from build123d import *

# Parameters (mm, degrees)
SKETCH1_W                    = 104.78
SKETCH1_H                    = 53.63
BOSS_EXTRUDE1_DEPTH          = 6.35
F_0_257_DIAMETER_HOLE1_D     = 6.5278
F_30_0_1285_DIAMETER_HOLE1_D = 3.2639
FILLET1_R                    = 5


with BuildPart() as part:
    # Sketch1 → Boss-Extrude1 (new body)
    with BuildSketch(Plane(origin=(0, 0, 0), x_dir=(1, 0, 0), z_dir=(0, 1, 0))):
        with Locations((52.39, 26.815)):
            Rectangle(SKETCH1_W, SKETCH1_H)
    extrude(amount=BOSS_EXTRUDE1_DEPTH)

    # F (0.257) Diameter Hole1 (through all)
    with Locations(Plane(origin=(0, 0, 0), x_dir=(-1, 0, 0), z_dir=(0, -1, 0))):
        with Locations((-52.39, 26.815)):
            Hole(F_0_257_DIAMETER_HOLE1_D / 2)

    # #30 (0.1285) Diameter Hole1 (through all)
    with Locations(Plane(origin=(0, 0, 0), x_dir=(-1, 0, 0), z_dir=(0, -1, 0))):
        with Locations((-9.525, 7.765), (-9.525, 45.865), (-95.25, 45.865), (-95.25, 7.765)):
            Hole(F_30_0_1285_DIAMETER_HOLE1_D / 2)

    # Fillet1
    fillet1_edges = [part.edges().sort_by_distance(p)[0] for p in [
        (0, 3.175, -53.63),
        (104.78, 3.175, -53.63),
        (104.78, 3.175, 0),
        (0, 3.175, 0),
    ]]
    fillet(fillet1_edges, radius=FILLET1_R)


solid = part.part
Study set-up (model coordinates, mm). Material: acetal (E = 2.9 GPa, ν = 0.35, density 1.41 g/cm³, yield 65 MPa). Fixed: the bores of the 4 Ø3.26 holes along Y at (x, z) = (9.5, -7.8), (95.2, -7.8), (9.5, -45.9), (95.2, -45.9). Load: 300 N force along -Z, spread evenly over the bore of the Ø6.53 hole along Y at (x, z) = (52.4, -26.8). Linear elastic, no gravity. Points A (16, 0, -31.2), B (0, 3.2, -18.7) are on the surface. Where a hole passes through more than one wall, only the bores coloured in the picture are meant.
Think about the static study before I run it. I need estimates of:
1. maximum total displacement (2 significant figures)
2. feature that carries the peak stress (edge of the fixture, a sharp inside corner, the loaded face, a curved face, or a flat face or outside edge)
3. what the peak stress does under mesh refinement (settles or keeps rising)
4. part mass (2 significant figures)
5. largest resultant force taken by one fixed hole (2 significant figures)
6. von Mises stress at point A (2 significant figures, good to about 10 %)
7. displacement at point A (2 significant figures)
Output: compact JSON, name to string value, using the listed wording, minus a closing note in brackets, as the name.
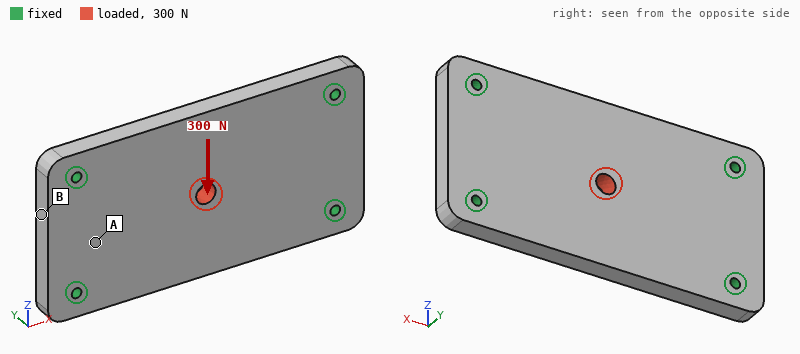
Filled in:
{"maximum total displacement": "30 µm", "feature that carries the peak stress": "edge of the fixture", "what the peak stress does under mesh refinement": "keeps rising", "part mass": "50 g", "largest resultant force taken by one fixed hole": "110 N", "von Mises stress at point A": "0.85 MPa", "displacement at point A": "5.2 µm"}
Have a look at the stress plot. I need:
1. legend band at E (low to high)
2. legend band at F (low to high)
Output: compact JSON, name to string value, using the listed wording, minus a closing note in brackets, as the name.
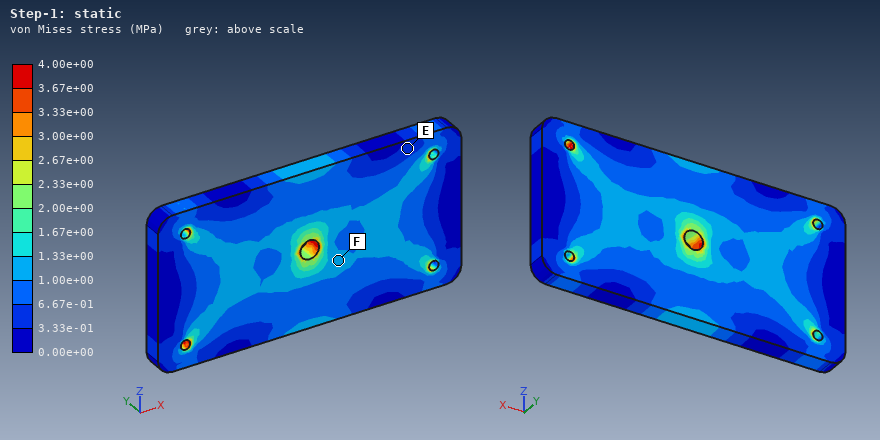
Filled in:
{"legend band at E": "3.33e-01 to 6.67e-01 MPa", "legend band at F": "1.00e+00 to 1.33e+00 MPa"}
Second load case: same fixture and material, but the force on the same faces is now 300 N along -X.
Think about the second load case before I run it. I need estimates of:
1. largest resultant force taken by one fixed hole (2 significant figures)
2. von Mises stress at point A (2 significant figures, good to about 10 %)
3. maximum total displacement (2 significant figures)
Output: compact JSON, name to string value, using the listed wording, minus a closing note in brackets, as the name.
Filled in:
{"largest resultant force taken by one fixed hole": "77 N", "von Mises stress at point A": "0.27 MPa", "maximum total displacement": "15 µm"}
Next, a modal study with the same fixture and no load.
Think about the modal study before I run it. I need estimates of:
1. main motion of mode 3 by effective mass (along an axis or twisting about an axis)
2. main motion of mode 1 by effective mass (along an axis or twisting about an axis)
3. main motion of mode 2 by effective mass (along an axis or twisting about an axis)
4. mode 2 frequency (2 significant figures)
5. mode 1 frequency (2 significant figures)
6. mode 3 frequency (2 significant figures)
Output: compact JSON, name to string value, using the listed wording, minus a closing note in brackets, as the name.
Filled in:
{"main motion of mode 3 by effective mass": "twisting about Z", "main motion of mode 1 by effective mass": "along Y", "main motion of mode 2 by effective mass": "twisting about X", "mode 2 frequency": "1700 Hz", "mode 1 frequency": "1100 Hz", "mode 3 frequency": "2900 Hz"}
